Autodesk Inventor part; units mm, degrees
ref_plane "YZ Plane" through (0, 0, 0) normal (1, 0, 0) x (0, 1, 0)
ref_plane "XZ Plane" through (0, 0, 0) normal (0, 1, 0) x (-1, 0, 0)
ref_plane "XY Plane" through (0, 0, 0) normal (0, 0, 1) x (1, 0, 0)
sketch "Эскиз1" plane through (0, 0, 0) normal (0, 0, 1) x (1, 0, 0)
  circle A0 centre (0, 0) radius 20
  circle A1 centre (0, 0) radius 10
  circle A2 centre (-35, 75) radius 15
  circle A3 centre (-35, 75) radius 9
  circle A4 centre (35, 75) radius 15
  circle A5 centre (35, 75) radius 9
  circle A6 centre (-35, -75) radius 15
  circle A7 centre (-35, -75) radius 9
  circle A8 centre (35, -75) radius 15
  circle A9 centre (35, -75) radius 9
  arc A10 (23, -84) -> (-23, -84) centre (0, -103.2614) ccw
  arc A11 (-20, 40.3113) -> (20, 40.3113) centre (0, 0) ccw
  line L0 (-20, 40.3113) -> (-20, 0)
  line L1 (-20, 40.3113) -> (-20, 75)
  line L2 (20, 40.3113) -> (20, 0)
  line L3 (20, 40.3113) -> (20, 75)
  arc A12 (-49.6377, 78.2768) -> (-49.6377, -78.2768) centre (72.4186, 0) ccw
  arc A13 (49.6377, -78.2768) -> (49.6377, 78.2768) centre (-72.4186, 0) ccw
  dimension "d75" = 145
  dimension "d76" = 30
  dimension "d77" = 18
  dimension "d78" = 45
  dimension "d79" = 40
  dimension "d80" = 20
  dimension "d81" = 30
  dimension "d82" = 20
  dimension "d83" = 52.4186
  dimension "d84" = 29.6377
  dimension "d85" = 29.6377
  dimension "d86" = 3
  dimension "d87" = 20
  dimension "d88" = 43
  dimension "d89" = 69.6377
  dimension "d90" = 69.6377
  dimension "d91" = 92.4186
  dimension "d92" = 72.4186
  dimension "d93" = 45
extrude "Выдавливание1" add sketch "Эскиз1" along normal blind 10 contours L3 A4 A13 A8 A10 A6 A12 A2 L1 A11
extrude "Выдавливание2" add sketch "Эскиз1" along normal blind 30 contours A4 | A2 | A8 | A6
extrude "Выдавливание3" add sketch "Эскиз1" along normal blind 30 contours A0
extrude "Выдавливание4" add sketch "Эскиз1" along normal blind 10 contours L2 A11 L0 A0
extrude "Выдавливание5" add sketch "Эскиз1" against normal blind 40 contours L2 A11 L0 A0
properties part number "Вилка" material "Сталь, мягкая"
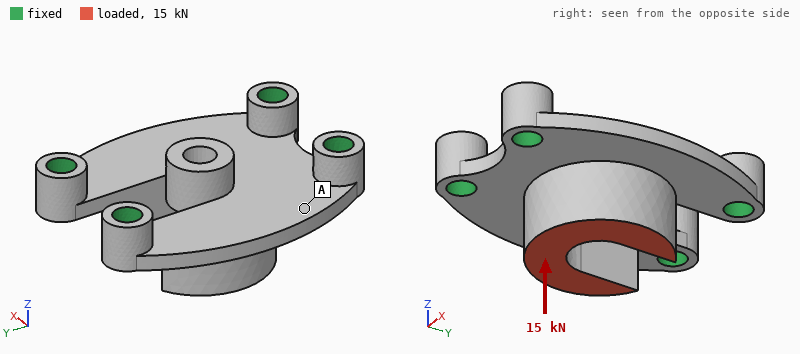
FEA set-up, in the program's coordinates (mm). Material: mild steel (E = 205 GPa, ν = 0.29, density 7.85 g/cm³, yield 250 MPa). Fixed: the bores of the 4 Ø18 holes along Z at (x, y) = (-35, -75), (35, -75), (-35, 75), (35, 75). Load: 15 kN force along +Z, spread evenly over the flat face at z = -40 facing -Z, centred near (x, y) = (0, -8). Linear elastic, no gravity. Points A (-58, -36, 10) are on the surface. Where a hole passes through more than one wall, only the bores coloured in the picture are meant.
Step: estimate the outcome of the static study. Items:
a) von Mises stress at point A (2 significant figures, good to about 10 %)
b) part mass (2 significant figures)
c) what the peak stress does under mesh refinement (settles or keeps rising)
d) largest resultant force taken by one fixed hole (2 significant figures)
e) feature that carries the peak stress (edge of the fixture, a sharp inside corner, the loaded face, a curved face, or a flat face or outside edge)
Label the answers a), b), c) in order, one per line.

a) 13 MPa
b) 3.1 kg
c) keeps rising
d) 5.0 kN
e) a sharp inside corner
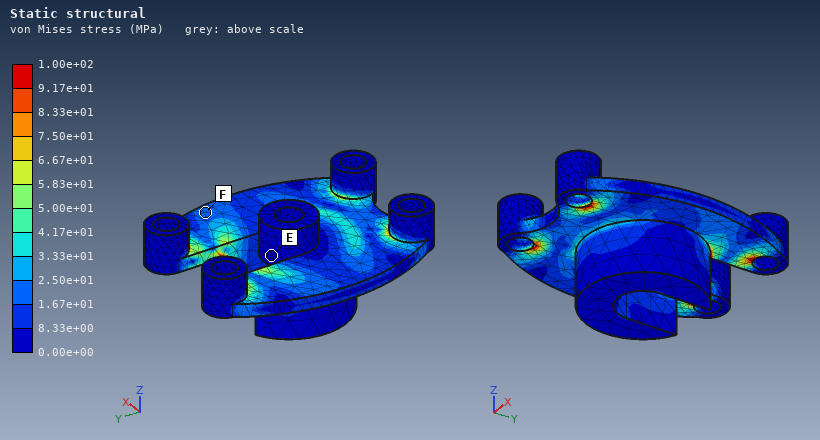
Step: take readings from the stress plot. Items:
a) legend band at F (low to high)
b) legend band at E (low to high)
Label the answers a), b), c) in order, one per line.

a) 1.67e+01 to 2.50e+01 MPa
b) 0.00e+00 to 8.33e+00 MPa
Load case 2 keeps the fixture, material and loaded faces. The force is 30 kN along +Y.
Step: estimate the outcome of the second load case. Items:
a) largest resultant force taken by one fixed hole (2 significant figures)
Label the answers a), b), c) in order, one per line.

a) 11 kN
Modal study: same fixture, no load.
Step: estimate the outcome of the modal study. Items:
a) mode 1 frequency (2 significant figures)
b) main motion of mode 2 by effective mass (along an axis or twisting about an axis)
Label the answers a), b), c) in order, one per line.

a) 2200 Hz
b) along Z
